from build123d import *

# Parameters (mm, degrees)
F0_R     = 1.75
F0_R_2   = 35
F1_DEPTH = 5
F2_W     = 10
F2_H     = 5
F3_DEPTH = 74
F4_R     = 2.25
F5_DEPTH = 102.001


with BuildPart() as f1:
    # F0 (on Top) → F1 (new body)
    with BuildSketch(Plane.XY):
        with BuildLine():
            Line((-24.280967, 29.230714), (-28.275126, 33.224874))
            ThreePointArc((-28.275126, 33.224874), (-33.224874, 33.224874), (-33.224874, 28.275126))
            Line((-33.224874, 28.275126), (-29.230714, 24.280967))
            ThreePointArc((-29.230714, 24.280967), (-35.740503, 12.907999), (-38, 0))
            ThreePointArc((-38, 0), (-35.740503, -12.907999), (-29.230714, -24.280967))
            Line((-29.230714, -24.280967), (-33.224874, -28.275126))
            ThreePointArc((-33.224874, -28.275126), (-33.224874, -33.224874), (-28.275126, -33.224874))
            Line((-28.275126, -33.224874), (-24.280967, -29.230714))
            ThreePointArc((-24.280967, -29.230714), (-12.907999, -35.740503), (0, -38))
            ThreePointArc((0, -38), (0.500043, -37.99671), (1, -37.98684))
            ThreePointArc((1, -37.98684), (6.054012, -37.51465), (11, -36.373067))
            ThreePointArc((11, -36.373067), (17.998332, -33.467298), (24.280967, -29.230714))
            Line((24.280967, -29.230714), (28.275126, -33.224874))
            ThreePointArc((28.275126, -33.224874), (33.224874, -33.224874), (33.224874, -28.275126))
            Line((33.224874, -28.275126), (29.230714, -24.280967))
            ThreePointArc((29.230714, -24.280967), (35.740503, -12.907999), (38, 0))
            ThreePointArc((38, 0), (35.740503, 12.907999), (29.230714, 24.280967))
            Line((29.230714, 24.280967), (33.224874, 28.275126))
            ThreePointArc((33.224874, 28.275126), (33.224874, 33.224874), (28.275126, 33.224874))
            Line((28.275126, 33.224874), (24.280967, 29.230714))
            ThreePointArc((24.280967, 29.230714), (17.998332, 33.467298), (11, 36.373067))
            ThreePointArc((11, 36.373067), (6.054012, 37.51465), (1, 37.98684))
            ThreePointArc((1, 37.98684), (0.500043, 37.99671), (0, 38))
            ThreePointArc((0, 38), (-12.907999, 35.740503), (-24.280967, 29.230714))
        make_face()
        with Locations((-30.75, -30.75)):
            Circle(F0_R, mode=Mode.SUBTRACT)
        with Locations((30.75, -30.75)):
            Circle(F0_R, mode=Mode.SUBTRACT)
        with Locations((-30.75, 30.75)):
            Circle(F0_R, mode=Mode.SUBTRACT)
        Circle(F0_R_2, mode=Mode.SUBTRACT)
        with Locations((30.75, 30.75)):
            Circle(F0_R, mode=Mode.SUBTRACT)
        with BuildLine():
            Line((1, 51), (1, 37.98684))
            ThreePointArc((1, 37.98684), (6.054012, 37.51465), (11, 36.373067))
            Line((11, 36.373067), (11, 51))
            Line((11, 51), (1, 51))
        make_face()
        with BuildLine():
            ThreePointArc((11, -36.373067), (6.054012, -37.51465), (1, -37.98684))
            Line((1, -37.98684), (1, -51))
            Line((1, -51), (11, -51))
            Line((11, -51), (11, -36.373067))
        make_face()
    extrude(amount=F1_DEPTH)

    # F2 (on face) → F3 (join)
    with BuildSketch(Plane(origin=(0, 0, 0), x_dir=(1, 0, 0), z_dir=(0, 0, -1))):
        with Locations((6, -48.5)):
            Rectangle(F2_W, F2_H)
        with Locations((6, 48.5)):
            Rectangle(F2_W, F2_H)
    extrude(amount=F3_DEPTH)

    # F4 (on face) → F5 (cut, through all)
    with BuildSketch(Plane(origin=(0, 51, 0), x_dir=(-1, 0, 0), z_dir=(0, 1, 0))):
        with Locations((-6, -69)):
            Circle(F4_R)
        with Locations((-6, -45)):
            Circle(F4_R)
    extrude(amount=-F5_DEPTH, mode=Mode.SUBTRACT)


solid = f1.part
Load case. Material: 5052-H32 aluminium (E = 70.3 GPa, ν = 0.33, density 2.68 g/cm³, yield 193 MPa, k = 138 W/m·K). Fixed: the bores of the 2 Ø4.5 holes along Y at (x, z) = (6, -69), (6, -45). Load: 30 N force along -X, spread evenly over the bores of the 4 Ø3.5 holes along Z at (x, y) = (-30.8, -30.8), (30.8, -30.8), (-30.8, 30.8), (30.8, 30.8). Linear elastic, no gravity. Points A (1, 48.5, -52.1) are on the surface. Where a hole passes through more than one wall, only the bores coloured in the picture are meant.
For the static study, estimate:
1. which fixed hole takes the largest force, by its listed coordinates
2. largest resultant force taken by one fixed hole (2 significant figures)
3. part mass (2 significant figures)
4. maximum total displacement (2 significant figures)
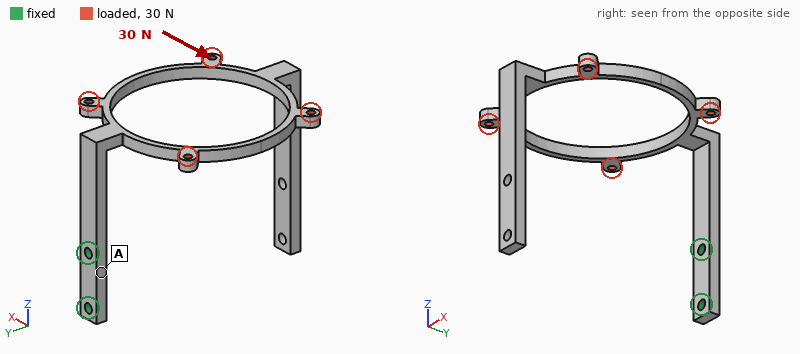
(6, -45)
44 N
34 g
1.7 mm
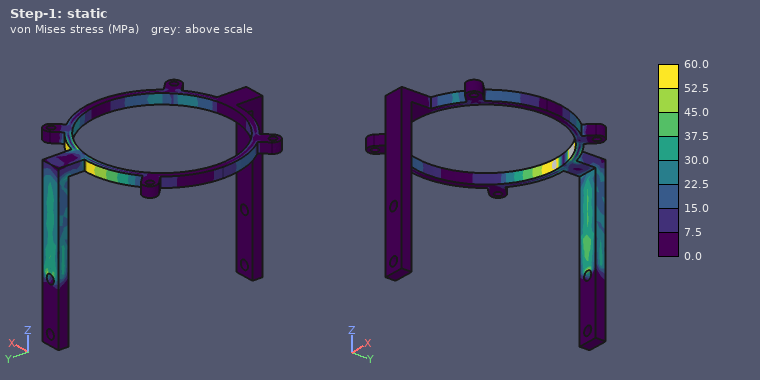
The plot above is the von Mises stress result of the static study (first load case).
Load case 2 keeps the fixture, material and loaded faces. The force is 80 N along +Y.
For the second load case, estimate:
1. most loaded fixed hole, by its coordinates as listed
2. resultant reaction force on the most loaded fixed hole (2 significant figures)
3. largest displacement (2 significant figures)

(6, -45)
85 N
1.5 mm
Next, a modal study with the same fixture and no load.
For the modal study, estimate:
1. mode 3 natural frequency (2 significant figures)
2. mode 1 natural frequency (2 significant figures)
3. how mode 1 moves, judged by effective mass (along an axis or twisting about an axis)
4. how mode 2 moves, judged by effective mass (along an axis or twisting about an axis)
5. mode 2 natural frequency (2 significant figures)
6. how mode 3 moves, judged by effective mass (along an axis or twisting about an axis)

250 Hz
87 Hz
along Z
along X
110 Hz
along Y
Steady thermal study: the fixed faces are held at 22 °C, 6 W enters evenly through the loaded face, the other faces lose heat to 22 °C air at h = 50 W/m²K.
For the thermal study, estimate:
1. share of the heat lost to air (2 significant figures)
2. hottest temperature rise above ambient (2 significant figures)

83 %
23 K
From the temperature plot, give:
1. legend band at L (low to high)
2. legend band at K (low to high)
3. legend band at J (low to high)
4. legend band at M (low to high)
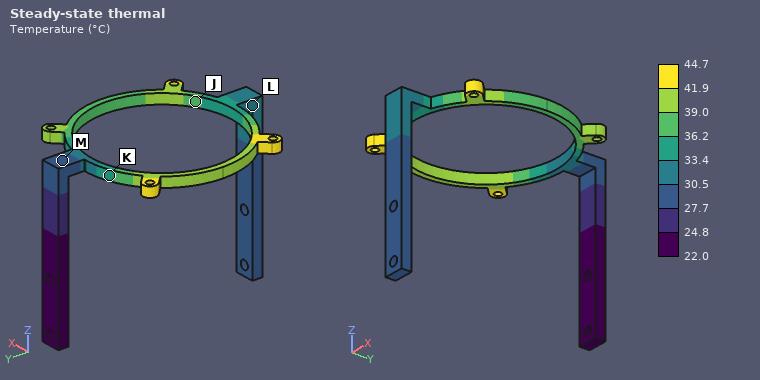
30.5 to 33.4 °C
33.4 to 36.2 °C
36.2 to 39.0 °C
27.7 to 30.5 °C
